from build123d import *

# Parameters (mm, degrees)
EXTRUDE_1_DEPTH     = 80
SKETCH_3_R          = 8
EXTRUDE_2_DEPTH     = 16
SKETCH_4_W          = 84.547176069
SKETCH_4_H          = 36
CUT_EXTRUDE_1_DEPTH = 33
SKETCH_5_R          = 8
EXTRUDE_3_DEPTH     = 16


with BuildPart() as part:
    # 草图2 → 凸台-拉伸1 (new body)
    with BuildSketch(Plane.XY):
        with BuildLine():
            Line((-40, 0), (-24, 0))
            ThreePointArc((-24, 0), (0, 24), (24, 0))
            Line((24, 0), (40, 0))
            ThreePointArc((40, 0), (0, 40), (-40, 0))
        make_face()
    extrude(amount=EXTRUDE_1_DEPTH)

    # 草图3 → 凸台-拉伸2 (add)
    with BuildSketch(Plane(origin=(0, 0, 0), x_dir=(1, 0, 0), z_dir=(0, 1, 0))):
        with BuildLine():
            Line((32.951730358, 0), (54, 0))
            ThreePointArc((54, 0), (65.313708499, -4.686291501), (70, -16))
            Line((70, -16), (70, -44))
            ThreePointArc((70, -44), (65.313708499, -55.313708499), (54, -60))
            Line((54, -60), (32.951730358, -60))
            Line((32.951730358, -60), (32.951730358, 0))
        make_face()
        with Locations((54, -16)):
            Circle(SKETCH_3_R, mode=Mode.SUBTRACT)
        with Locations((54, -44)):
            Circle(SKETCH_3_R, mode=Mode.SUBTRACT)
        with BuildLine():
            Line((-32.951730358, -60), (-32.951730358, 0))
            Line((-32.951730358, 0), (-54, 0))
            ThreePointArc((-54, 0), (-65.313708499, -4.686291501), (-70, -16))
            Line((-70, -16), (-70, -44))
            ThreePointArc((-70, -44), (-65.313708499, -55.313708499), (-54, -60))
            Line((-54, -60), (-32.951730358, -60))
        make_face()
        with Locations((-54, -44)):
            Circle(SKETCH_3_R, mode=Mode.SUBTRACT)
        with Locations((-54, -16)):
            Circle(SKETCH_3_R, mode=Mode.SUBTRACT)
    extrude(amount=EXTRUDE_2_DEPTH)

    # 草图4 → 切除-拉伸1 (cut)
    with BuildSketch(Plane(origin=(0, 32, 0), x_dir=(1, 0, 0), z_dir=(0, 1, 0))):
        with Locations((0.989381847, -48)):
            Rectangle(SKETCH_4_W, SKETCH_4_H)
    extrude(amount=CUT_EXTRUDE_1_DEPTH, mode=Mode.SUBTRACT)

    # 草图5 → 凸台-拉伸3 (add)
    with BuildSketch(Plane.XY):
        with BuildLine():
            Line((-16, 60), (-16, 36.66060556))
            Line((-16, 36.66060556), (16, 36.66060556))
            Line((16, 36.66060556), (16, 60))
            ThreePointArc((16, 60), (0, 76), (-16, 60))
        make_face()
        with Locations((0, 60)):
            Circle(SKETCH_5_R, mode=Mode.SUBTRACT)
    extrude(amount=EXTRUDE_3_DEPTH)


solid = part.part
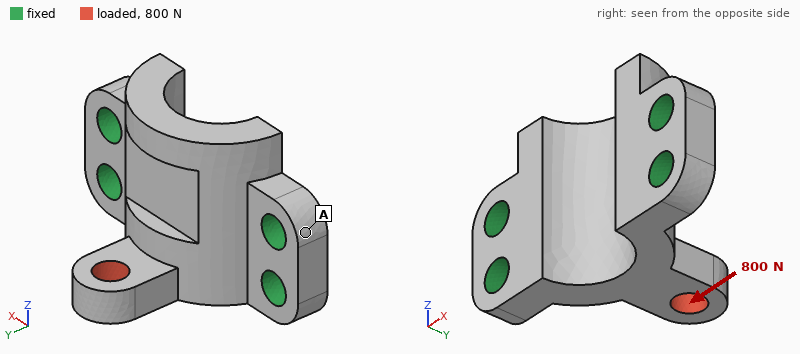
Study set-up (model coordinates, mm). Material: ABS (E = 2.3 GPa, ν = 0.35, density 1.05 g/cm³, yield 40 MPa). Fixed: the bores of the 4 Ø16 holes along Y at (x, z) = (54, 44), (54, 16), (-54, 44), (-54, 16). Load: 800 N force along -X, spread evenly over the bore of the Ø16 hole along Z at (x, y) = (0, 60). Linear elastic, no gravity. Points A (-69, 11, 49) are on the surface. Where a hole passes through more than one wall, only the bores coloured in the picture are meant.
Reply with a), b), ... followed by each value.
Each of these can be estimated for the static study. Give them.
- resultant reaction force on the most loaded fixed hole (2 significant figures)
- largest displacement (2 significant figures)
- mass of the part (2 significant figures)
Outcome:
a) 450 N
b) 0.38 mm
c) 190 g
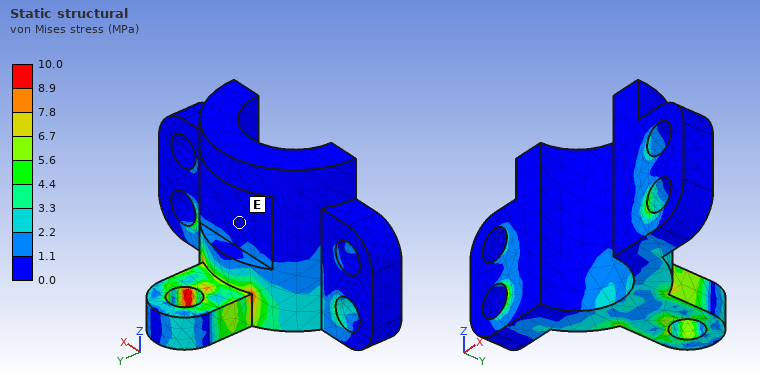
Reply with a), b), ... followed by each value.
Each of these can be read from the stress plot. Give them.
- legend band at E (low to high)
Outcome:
a) 0.0 to 1.1 MPa
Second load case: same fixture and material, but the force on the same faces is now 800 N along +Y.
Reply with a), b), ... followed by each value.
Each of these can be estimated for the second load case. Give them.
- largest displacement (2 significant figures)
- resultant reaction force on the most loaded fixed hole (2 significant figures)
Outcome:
a) 0.20 mm
b) 560 N
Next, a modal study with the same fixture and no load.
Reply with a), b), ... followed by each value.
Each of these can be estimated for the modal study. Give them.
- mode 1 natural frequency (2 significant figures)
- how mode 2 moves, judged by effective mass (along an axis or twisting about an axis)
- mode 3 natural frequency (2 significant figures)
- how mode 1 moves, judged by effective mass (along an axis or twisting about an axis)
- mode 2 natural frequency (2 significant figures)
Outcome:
a) 1300 Hz
b) along Y
c) 2400 Hz
d) along Z
e) 2100 Hz
